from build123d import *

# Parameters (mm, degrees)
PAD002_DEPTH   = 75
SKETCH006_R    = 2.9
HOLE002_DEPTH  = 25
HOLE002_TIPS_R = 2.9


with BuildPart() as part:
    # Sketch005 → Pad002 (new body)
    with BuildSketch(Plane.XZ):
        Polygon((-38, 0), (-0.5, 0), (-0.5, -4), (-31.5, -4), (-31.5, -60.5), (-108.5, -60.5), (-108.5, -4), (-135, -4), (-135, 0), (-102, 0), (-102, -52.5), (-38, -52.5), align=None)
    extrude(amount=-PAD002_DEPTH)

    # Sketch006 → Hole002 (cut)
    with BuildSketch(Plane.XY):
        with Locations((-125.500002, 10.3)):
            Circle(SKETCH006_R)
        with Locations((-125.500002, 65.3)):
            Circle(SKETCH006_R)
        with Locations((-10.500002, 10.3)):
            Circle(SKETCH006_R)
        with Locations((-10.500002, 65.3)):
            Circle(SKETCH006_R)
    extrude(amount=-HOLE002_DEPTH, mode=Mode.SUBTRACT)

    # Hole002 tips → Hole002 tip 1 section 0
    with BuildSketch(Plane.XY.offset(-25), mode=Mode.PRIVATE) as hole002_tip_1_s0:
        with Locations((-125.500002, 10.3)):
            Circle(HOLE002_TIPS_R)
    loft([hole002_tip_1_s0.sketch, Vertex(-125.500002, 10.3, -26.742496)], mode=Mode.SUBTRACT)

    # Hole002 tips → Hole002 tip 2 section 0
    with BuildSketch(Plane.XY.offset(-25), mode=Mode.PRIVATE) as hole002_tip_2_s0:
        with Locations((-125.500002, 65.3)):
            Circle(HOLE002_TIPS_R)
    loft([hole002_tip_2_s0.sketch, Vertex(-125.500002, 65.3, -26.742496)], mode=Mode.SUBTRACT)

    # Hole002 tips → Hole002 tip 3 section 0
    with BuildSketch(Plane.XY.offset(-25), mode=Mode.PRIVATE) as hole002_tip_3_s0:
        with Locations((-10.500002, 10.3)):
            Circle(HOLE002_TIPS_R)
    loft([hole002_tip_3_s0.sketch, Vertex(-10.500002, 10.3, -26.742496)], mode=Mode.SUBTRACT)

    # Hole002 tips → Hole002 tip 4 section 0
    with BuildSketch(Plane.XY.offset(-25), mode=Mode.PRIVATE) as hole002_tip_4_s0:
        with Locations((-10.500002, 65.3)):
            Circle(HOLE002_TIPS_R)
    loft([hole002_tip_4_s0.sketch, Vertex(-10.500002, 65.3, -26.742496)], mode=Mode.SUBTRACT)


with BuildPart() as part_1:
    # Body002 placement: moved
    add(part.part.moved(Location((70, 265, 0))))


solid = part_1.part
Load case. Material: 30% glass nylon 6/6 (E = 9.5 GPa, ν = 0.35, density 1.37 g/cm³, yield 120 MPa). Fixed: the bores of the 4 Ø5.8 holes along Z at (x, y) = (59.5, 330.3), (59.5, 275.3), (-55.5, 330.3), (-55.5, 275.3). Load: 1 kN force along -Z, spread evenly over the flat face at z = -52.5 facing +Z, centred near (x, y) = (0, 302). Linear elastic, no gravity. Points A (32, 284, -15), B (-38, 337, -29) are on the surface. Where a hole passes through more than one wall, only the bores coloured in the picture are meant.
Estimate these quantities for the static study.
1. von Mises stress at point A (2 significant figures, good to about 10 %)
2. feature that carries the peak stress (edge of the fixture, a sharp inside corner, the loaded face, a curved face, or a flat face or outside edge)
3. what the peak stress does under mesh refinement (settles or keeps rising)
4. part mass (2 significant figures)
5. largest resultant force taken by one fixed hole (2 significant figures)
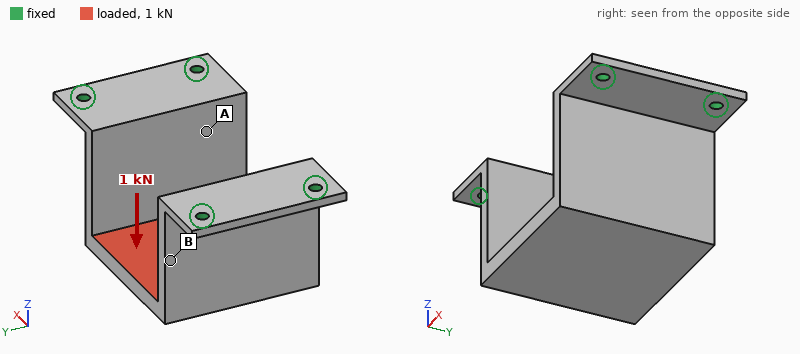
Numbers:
5.1 MPa
edge of the fixture
keeps rising
160 g
280 N
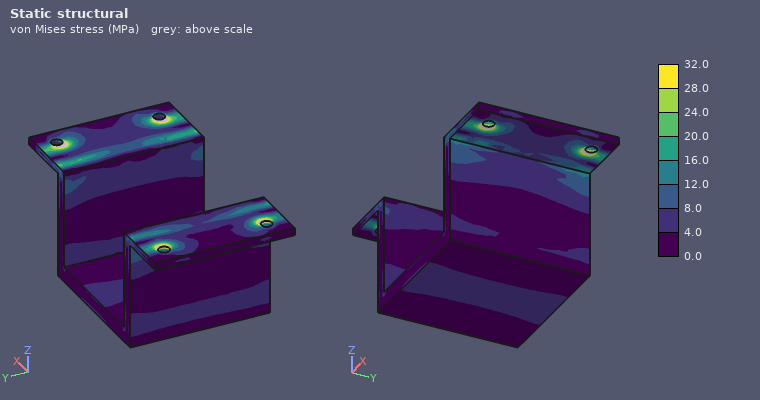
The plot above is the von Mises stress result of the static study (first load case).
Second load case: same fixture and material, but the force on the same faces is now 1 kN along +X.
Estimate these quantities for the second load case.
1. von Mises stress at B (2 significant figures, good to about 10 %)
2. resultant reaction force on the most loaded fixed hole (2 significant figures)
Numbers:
8.7 MPa
350 N
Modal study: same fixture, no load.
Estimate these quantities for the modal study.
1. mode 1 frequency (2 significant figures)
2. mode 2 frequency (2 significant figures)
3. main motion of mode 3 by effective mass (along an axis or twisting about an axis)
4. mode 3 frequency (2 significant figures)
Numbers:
560 Hz
580 Hz
twisting about Z
910 Hz
